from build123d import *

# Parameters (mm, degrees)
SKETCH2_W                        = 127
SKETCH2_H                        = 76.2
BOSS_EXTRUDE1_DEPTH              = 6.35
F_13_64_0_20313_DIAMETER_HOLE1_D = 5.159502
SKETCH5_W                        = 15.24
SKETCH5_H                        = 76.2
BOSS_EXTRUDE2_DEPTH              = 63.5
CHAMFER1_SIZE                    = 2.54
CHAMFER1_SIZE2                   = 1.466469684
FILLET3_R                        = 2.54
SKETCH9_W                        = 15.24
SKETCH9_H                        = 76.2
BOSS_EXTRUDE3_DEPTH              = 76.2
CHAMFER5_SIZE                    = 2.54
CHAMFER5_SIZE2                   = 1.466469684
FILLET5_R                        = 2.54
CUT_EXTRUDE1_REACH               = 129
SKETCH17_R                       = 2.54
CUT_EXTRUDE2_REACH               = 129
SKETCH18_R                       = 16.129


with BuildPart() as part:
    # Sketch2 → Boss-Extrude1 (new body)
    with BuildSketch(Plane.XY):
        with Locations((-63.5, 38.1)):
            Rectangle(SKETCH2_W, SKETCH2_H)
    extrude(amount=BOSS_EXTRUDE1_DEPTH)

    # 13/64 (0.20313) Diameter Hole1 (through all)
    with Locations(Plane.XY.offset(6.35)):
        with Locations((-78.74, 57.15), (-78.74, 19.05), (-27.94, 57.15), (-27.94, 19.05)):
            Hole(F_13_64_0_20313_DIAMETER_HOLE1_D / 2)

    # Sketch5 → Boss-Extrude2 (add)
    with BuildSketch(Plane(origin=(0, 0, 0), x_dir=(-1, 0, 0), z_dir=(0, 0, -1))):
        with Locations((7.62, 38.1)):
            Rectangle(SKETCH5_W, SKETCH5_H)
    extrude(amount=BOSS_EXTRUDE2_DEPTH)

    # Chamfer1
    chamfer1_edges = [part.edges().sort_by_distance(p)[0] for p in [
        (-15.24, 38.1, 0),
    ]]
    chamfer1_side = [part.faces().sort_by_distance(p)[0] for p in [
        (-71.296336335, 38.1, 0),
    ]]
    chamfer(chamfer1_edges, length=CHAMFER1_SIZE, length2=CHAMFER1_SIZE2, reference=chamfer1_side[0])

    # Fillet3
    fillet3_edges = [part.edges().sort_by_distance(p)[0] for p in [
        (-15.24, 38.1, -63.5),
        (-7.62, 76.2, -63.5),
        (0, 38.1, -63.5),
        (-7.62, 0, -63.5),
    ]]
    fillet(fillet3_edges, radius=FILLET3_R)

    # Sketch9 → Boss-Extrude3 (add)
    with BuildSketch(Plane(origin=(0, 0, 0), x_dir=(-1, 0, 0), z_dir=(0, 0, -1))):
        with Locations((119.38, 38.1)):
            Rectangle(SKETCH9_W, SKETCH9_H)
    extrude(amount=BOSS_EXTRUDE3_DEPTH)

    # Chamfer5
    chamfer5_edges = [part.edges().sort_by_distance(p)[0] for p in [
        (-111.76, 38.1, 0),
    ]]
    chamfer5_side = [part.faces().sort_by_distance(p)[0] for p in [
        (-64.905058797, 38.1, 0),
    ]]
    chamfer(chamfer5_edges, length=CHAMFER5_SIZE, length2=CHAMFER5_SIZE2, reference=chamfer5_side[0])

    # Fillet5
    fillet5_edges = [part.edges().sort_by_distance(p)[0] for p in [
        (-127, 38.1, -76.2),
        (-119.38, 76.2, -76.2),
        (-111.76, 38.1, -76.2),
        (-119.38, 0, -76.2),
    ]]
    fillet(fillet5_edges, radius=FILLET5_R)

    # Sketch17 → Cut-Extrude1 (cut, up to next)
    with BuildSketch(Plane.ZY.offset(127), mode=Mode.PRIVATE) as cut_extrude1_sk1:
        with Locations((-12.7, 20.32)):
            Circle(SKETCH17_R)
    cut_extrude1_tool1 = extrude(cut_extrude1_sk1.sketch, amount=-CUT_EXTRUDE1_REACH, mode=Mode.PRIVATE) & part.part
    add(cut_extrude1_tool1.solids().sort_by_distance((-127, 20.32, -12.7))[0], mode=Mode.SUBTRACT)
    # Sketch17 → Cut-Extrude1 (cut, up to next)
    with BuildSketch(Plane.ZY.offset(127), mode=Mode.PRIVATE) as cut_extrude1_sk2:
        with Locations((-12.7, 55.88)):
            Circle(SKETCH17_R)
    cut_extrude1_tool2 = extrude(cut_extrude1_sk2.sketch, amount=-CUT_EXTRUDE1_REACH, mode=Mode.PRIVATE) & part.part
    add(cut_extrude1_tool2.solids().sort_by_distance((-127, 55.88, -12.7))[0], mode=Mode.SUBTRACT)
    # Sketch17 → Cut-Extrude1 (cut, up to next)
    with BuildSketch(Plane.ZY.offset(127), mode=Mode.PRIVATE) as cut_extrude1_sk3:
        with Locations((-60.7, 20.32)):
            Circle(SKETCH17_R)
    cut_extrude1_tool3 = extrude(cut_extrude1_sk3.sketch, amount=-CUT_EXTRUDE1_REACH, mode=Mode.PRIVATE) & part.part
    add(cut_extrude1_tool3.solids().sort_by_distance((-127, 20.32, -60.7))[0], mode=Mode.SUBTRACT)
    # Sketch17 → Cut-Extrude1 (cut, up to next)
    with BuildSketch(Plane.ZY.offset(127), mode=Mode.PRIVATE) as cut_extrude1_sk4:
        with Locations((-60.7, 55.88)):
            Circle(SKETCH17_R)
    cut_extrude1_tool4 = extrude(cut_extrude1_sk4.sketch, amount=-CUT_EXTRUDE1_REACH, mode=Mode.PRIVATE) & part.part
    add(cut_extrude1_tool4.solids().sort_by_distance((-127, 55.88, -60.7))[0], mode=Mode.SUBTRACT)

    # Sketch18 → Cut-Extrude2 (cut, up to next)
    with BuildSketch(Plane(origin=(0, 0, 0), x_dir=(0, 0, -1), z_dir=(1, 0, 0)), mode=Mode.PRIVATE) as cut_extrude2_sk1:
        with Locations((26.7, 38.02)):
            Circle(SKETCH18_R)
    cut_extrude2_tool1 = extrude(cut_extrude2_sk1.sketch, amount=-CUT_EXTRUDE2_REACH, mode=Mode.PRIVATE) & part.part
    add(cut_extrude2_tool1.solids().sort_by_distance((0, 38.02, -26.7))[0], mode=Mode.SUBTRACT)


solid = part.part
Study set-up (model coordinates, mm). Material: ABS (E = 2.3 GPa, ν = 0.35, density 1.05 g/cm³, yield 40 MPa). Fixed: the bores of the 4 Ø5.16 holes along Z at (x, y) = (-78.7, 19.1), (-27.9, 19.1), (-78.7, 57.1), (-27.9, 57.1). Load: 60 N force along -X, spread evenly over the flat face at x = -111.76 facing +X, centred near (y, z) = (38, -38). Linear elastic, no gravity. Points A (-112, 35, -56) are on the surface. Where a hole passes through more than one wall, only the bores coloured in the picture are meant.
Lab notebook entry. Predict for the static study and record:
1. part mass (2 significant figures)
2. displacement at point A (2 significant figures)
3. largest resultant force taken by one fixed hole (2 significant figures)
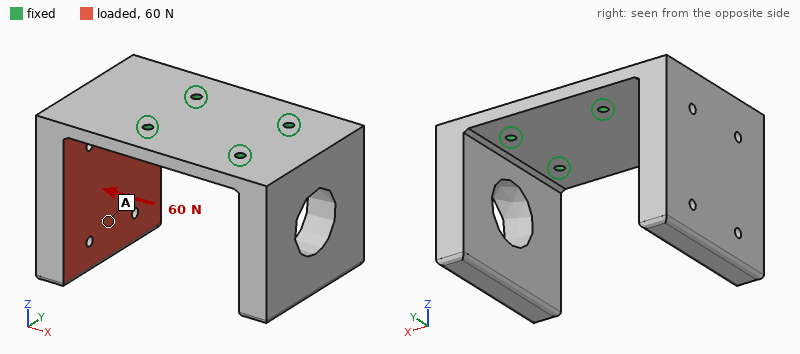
220 g
1.4 mm
27 N
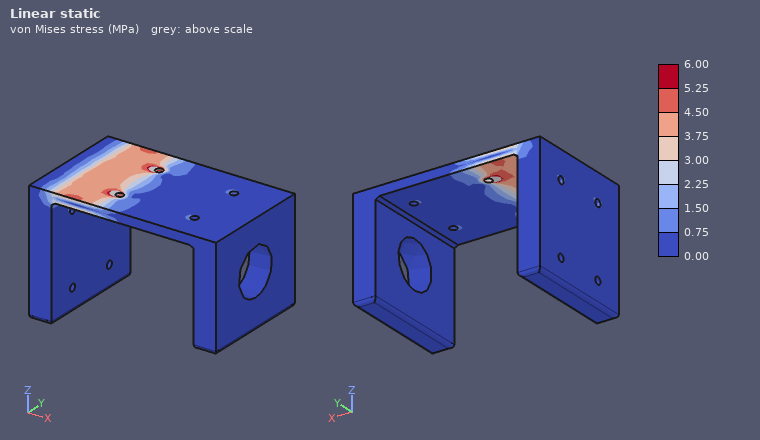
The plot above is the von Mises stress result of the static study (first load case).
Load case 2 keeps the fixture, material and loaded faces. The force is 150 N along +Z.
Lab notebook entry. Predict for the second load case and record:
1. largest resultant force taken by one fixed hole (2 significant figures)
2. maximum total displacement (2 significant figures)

89 N
1.9 mm
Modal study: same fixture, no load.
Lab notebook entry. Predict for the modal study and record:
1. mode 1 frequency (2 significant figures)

100 Hz
